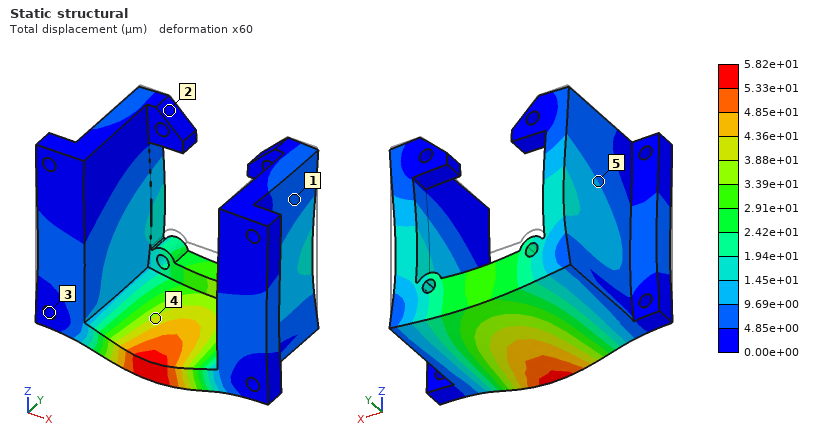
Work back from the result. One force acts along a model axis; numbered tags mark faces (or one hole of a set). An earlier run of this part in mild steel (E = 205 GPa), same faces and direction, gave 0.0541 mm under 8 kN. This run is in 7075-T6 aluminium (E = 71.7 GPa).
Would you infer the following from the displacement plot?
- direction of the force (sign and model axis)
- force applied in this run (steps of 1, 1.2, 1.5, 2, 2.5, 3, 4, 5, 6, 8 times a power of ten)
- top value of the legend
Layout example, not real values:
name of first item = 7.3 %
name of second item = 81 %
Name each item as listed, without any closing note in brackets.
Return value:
direction of the force = -Z
force applied in this run = 3 kN
top value of the legend = 5.82e+01 µm
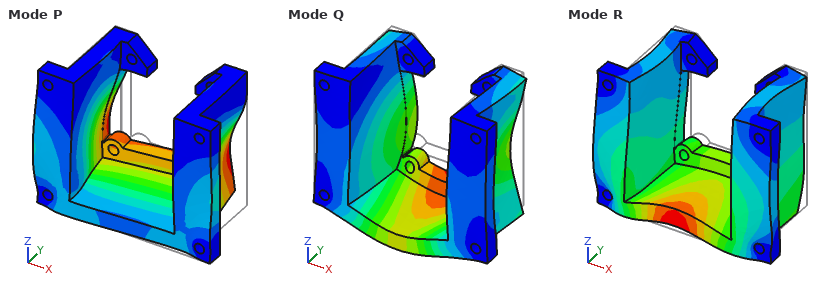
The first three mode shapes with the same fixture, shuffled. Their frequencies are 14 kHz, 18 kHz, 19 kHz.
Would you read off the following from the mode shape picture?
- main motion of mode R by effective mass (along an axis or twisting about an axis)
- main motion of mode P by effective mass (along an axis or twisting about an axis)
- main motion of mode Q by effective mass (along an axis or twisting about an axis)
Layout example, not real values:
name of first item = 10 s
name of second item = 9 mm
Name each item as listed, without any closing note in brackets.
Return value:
main motion of mode R by effective mass = along Y
main motion of mode P by effective mass = along X
main motion of mode Q by effective mass = along Z
